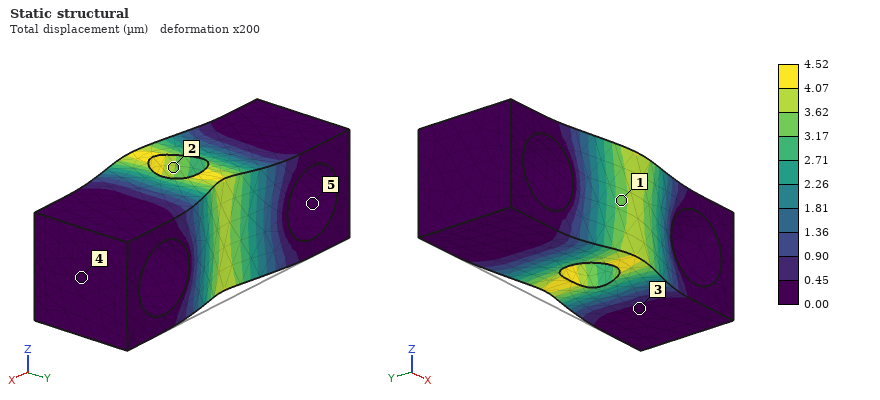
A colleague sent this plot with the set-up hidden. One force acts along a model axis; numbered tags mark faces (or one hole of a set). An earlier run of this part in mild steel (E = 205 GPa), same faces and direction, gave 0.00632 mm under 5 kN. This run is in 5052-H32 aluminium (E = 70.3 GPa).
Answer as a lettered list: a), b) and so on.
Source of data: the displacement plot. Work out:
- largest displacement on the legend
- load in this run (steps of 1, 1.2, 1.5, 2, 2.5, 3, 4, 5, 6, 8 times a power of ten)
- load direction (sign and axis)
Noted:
a) 4.52 µm
b) 1.2 kN
c) -Y
